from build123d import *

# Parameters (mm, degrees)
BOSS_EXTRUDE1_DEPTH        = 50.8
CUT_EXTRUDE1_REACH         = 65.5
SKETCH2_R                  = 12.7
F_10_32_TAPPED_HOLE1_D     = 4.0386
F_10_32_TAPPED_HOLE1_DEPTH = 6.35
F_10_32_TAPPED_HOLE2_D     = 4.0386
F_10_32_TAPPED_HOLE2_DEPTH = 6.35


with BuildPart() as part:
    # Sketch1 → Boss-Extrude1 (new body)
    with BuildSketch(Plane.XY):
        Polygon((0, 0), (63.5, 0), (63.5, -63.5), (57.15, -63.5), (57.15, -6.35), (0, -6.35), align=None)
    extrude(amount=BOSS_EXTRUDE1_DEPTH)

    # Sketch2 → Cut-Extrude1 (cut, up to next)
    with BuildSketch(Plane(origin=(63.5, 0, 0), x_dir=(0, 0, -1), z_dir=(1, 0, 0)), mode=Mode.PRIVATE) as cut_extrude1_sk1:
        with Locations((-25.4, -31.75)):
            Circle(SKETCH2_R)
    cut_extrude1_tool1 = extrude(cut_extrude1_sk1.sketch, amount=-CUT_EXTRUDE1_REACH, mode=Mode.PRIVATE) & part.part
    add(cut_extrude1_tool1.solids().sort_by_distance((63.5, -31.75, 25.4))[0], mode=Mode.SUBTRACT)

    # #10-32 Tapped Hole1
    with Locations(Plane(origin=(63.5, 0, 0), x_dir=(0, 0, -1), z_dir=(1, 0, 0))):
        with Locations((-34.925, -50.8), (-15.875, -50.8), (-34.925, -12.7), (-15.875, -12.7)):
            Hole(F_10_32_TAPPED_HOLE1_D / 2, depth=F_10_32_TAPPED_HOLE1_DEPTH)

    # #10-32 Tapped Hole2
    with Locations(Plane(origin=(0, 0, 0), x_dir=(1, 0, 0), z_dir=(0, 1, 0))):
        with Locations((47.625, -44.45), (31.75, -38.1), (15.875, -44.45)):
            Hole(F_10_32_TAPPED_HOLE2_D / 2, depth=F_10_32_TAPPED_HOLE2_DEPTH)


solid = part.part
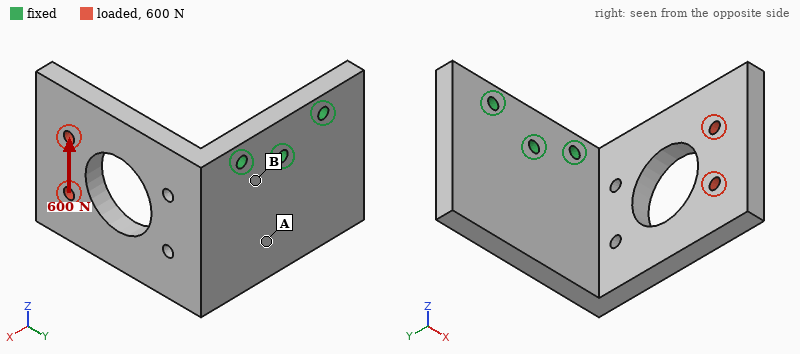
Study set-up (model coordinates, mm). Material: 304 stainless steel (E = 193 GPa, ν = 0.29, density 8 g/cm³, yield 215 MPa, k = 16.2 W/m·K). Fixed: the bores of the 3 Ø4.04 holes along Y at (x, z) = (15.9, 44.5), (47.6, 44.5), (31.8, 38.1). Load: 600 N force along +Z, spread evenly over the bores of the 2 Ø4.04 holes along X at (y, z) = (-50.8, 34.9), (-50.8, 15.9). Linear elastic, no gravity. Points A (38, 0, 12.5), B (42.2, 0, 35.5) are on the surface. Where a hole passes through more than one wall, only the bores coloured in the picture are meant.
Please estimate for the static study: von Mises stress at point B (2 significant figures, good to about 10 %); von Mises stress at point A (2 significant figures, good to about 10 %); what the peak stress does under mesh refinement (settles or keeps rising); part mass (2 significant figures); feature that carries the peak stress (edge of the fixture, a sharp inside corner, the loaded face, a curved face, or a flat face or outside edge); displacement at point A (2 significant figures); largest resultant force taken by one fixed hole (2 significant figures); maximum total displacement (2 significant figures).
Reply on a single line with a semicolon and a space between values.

53 MPa; 25 MPa; keeps rising; 280 g; edge of the fixture; 0.029 mm; 850 N; 0.14 mm
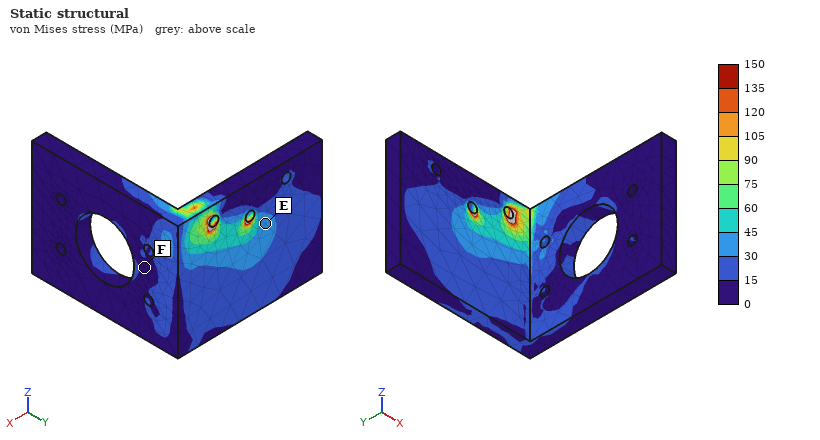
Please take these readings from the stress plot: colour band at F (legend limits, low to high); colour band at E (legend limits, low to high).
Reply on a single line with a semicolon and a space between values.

0 to 15 MPa; 30 to 45 MPa
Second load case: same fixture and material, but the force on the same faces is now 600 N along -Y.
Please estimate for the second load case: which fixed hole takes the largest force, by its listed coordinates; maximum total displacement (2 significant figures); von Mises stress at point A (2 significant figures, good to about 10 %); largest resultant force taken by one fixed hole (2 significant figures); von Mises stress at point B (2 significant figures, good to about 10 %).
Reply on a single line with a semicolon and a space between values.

(47.6, 44.5); 66 µm; 13 MPa; 560 N; 27 MPa
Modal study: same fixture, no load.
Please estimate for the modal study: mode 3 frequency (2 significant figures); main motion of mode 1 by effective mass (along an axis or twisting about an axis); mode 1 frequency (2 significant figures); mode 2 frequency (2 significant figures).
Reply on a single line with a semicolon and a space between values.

2900 Hz; along X; 900 Hz; 1300 Hz
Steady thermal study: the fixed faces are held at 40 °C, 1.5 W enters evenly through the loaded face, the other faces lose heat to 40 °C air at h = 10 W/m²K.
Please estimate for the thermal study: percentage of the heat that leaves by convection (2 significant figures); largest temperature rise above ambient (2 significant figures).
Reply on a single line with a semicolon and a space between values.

54 %; 18 K
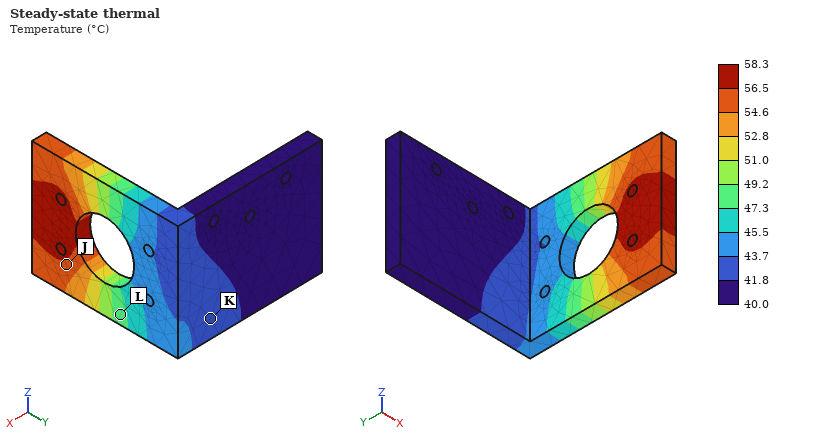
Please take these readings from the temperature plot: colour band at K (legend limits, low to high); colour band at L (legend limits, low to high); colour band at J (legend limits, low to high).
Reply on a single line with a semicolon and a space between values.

41.8 to 43.7 °C; 47.3 to 49.2 °C; 54.6 to 56.5 °C
